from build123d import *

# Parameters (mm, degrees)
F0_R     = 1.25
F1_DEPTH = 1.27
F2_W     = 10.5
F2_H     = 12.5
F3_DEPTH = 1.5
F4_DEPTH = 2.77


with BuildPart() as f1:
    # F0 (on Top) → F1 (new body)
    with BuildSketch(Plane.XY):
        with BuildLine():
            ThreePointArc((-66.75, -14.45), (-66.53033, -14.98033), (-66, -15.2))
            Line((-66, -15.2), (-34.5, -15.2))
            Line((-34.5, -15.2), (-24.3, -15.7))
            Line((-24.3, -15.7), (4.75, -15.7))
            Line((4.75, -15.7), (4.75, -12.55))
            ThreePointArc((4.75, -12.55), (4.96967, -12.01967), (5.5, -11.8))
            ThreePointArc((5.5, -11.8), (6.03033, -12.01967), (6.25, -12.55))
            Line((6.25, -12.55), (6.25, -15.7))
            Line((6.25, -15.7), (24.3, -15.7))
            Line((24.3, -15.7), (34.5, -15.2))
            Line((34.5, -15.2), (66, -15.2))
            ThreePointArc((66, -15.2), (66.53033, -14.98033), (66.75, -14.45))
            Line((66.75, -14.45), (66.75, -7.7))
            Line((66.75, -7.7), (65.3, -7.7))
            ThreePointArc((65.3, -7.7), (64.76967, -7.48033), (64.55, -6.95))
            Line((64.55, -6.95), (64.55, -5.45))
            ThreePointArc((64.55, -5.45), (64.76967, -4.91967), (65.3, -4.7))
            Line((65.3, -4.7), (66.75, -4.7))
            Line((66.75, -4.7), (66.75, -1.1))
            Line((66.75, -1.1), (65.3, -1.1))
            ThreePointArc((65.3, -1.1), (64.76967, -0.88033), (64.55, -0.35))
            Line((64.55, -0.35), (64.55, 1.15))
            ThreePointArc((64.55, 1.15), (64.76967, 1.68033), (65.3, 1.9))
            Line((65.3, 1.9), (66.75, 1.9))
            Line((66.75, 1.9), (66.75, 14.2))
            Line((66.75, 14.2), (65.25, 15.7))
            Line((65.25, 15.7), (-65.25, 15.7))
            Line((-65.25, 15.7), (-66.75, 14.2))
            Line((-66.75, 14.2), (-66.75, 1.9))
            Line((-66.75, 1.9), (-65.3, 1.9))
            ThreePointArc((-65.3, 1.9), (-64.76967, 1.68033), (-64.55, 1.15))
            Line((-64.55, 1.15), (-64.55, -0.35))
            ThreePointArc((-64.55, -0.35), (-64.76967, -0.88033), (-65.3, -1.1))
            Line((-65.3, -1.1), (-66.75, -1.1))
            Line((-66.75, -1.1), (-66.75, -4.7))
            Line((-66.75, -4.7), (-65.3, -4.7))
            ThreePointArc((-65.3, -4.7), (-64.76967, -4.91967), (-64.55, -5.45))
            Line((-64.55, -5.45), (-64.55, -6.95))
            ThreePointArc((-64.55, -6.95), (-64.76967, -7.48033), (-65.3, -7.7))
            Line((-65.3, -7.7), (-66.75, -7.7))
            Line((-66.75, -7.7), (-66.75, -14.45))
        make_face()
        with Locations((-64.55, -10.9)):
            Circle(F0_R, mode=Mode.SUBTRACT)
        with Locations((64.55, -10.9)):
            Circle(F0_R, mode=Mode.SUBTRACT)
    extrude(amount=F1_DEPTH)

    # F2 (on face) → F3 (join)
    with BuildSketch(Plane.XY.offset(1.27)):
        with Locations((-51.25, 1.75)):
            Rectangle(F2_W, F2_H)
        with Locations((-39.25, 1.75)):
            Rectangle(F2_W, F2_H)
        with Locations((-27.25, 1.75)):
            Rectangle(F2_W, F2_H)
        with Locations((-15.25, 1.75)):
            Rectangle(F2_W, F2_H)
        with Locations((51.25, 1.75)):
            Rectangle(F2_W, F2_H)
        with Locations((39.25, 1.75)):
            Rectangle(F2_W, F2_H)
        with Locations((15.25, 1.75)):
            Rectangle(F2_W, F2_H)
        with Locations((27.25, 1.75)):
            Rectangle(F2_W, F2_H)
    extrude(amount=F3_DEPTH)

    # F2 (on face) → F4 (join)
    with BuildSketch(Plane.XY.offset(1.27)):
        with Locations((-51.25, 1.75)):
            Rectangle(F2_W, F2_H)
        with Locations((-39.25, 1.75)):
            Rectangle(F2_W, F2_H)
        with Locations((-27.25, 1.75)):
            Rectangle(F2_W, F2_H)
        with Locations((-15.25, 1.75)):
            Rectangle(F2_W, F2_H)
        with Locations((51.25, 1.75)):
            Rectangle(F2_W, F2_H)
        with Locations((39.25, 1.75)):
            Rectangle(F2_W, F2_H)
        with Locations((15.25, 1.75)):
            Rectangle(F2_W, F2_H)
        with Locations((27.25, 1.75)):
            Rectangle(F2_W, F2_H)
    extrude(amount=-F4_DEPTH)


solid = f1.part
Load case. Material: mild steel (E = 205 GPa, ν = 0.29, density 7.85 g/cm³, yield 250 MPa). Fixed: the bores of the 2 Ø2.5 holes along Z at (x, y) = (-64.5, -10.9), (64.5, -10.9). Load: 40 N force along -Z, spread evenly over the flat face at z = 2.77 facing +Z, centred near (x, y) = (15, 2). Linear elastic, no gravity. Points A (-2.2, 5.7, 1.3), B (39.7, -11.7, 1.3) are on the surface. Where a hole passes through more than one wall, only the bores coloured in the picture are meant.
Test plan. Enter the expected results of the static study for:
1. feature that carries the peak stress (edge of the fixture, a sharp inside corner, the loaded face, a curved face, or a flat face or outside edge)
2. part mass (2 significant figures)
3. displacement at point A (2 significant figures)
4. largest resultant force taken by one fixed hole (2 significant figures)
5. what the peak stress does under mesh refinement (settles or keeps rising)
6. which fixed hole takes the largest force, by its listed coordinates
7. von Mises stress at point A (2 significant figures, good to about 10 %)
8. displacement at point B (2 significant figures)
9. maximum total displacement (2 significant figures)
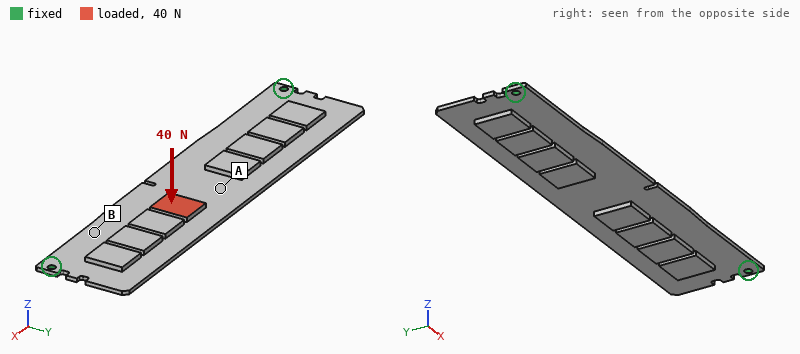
edge of the fixture
66 g
0.46 mm
26 N
keeps rising
(64.5, -10.9)
58 MPa
0.16 mm
0.52 mm
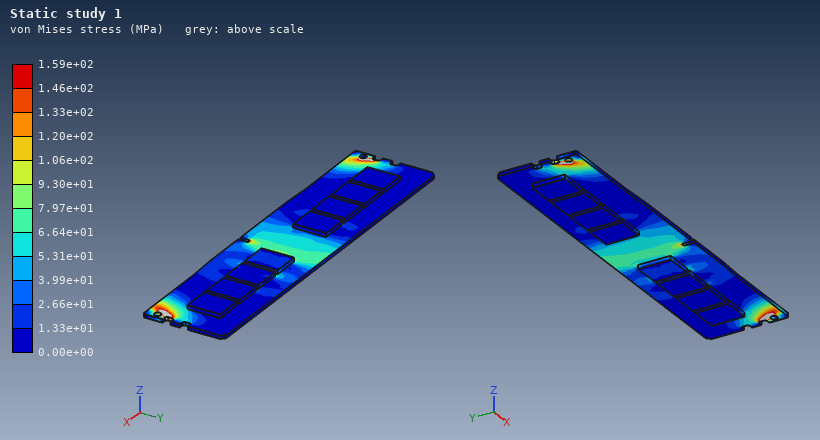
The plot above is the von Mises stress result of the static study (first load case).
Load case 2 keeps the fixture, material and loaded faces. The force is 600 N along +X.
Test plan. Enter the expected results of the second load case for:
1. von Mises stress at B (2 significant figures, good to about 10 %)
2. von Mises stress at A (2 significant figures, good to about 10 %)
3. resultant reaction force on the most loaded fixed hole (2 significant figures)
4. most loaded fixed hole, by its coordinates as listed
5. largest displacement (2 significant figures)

26 MPa
62 MPa
330 N
(64.5, -10.9)
0.24 mm
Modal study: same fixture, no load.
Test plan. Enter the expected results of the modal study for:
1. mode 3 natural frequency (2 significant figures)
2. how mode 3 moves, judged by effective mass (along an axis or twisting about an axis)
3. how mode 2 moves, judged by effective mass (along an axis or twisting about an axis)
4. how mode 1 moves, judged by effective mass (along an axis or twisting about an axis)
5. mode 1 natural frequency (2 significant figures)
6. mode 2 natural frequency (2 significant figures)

950 Hz
twisting about Y
twisting about X
along Z
270 Hz
820 Hz
